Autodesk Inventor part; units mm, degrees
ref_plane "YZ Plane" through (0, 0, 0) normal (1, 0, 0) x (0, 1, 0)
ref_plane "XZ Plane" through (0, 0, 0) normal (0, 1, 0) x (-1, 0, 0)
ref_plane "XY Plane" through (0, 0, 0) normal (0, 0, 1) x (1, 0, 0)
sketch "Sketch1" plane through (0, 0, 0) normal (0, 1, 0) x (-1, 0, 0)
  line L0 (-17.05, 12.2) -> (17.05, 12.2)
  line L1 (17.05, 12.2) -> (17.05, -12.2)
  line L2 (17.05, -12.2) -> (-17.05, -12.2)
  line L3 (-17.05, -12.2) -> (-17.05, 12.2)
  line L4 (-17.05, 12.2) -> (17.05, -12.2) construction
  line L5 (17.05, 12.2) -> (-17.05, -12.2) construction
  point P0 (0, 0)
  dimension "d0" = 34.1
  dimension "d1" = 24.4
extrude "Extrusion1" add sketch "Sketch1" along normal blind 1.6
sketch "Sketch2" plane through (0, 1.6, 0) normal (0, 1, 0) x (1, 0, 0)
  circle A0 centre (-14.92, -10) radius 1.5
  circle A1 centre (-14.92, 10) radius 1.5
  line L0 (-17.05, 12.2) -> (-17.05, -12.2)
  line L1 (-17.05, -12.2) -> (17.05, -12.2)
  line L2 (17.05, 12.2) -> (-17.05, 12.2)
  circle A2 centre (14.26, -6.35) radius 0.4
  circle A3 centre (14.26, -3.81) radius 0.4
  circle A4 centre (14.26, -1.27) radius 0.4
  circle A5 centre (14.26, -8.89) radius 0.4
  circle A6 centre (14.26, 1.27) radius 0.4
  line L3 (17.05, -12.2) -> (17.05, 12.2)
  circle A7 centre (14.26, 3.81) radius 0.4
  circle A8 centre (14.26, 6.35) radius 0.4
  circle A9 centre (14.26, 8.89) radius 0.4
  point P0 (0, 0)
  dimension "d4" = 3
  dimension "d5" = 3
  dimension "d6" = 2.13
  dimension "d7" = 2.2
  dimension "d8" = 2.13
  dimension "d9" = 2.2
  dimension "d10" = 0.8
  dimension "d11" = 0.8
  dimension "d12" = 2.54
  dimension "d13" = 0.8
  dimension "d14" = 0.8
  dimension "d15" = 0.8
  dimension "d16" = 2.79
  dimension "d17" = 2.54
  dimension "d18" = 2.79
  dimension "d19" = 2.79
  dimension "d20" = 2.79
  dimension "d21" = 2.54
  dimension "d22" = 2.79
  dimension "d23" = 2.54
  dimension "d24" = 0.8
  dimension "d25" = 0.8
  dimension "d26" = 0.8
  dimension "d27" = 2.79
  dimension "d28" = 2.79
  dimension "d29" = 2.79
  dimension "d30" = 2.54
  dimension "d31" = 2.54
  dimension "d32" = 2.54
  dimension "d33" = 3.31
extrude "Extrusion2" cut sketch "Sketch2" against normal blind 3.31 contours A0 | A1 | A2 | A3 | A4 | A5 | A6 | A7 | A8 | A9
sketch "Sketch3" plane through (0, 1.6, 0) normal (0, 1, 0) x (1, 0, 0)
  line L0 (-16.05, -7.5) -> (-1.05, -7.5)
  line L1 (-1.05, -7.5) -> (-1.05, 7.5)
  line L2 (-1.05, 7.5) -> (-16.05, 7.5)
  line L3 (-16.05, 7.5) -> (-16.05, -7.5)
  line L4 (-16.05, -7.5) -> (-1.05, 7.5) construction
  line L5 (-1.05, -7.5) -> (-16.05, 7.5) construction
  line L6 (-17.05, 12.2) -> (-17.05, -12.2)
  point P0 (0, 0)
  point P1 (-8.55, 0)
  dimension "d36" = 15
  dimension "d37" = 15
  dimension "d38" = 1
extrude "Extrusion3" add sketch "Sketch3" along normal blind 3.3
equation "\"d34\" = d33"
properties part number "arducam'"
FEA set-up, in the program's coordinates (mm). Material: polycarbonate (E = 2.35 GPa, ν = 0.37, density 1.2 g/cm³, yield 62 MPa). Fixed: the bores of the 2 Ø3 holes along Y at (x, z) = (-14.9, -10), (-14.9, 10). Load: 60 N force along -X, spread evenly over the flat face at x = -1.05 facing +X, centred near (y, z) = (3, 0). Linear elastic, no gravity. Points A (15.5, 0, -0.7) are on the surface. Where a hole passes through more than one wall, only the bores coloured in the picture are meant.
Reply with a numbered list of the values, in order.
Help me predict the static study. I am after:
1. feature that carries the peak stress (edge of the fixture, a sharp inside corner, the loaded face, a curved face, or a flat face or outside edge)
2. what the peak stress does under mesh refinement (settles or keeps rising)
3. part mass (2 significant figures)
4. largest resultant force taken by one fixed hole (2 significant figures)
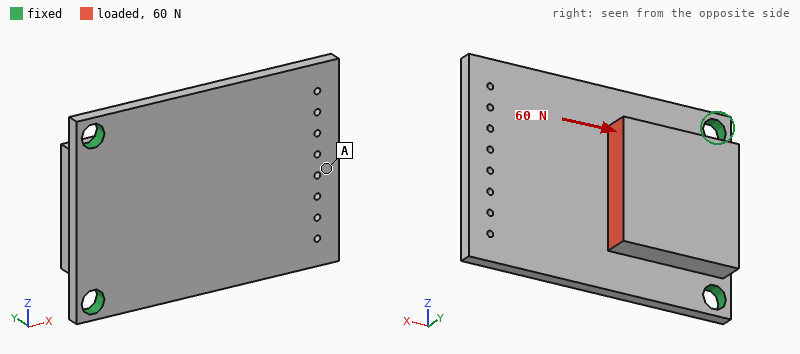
1. edge of the fixture
2. keeps rising
3. 2.5 g
4. 31 N
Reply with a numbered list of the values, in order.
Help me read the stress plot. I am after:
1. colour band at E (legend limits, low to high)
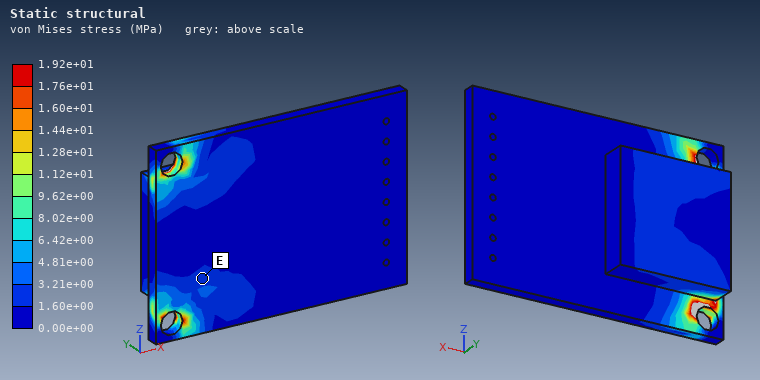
1. 1.60e+00 to 3.21e+00 MPa
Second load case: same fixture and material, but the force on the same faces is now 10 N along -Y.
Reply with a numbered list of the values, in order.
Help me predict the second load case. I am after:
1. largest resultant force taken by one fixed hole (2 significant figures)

1. 5.6 N
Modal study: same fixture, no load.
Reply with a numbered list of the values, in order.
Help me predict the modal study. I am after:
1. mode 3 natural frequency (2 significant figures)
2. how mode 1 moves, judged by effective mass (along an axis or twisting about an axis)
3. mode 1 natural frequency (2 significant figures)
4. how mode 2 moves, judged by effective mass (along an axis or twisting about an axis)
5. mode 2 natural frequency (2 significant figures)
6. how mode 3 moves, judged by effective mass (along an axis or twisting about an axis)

1. 2200 Hz
2. along Y
3. 580 Hz
4. twisting about X
5. 1700 Hz
6. along Y
